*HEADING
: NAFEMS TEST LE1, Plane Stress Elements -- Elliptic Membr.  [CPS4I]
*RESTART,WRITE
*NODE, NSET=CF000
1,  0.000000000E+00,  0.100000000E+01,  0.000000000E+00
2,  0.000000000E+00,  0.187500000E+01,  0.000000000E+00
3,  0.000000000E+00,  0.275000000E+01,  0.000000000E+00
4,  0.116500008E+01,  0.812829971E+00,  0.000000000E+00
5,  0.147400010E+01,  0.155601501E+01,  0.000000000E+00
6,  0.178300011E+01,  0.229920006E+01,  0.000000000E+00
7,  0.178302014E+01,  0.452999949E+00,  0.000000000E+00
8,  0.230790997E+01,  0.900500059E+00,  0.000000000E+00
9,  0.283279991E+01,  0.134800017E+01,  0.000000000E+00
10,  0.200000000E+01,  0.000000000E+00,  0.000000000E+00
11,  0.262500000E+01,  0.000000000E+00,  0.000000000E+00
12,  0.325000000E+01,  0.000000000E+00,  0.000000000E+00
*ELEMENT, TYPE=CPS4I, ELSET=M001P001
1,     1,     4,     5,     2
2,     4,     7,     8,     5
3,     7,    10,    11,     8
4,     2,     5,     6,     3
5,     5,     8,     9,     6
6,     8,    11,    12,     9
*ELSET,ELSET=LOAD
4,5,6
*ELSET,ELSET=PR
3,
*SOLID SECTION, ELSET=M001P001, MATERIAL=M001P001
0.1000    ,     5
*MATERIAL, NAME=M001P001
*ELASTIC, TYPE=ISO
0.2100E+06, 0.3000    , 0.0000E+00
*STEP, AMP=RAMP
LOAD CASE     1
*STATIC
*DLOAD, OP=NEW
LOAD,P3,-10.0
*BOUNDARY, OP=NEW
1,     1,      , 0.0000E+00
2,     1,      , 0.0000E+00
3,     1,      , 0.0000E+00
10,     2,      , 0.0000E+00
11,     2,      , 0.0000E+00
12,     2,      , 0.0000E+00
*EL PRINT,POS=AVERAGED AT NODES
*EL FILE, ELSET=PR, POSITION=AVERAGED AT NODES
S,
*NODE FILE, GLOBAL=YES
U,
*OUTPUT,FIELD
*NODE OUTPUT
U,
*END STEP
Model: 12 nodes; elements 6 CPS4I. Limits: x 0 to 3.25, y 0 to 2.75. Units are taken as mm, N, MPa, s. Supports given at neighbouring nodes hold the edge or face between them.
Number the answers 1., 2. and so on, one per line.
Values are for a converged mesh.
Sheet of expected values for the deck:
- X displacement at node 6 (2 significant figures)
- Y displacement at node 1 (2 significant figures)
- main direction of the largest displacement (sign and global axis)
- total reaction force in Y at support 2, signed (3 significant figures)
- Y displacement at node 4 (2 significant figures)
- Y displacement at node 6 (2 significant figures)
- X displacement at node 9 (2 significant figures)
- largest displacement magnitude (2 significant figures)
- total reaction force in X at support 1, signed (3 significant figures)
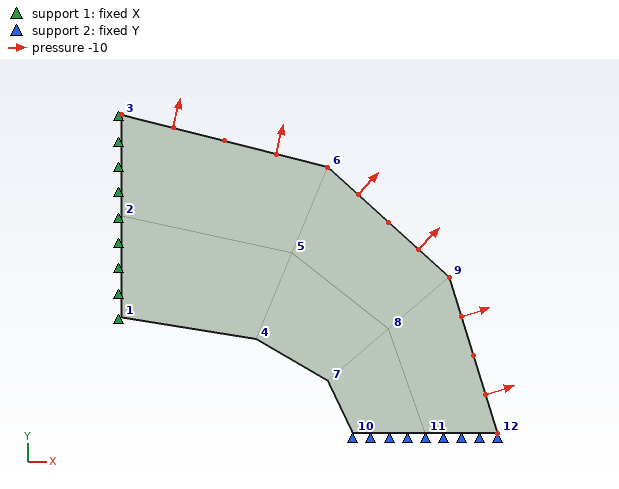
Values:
1. 1.9e-04 mm
2. 5.5e-04 mm
3. +Y
4. -3.25 N
5. 4.1e-04 mm
6. 3.2e-04 mm
7. 7.4e-05 mm
8. 5.6e-04 mm
9. -2.75 N
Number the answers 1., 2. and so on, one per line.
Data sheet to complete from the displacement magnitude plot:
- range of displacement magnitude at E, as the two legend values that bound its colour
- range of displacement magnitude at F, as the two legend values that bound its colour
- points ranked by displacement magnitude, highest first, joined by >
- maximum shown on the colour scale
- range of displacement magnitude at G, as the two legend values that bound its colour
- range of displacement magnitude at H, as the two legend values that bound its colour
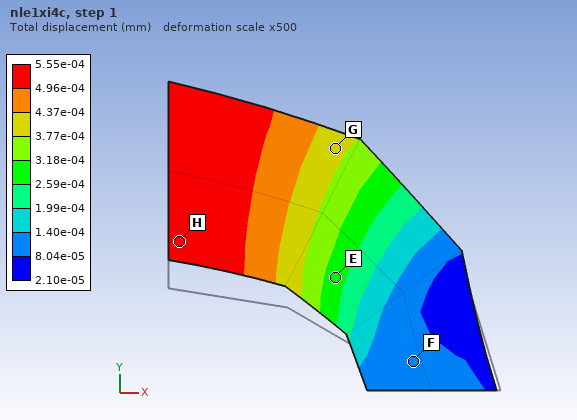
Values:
1. 2.59e-04 to 3.18e-04 mm
2. 8.04e-05 to 1.40e-04 mm
3. H > G > E > F
4. 5.55e-04 mm
5. 3.77e-04 to 4.37e-04 mm
6. 4.96e-04 to 5.55e-04 mm
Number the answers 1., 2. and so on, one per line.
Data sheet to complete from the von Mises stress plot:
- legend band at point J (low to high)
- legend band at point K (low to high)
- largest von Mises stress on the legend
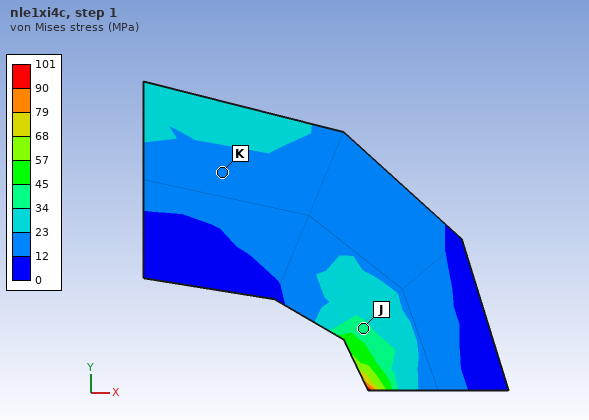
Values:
1. 34 to 45 MPa
2. 12 to 23 MPa
3. 101 MPa
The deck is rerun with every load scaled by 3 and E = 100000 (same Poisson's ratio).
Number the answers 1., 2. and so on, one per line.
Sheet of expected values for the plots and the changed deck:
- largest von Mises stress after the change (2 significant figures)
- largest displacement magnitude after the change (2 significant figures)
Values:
1. 300 MPa
2. 0.0035 mm
